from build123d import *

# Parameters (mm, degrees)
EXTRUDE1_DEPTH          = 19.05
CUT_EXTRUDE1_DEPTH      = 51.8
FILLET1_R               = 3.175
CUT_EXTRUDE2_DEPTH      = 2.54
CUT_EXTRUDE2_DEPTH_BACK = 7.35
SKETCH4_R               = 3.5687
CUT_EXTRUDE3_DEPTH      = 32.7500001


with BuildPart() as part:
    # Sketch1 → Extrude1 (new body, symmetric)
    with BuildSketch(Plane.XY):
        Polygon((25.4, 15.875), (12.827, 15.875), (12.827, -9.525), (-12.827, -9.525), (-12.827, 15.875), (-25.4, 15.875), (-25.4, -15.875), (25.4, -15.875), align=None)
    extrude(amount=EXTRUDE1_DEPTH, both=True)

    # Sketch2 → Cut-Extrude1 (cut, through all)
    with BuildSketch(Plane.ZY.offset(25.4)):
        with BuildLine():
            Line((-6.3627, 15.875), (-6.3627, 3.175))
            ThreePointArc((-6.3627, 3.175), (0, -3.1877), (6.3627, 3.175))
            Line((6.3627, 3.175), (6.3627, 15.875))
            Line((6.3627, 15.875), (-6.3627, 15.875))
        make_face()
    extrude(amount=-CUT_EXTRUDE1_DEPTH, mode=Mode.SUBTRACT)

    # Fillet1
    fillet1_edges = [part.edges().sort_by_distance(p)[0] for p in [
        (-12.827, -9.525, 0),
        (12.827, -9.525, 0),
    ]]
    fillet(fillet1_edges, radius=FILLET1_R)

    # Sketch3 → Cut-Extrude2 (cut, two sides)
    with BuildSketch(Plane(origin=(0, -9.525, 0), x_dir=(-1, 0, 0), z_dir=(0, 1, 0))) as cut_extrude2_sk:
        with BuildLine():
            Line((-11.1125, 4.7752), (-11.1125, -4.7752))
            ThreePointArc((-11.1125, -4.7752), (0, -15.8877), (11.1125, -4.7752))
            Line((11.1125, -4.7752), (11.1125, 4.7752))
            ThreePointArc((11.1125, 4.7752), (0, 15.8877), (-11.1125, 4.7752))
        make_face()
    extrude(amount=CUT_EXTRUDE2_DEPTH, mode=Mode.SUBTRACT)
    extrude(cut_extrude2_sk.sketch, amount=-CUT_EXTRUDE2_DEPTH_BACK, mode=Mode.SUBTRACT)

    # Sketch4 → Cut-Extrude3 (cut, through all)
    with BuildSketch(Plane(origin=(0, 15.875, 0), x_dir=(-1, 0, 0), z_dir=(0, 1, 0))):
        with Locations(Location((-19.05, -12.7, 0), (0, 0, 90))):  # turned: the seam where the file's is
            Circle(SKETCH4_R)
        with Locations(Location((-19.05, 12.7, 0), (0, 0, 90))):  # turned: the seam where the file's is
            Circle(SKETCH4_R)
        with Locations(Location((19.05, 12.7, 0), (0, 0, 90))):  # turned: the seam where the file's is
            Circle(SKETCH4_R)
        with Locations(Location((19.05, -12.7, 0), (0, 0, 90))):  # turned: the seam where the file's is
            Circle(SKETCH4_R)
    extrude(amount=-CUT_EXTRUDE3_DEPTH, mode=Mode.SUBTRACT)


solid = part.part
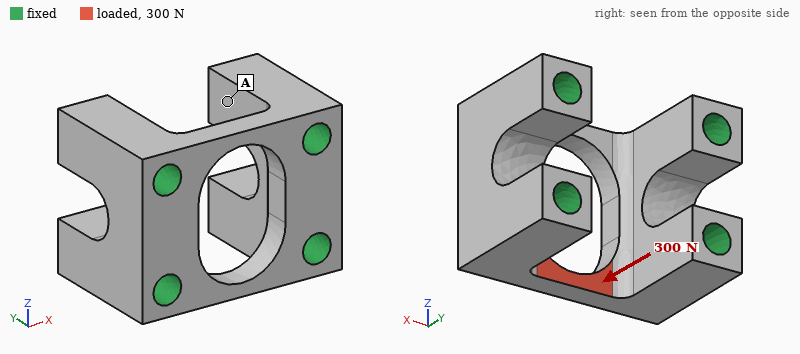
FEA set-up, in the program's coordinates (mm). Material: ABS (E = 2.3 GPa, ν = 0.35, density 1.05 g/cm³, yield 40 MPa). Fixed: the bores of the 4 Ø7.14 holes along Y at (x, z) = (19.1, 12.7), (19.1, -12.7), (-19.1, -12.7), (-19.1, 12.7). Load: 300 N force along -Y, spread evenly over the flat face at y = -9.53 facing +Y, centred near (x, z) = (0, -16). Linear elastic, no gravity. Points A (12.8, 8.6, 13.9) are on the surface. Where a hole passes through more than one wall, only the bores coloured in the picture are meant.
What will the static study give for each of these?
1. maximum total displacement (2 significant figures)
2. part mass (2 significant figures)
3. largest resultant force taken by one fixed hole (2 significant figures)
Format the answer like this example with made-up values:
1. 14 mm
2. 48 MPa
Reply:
1. 0.13 mm
2. 23 g
3. 150 N
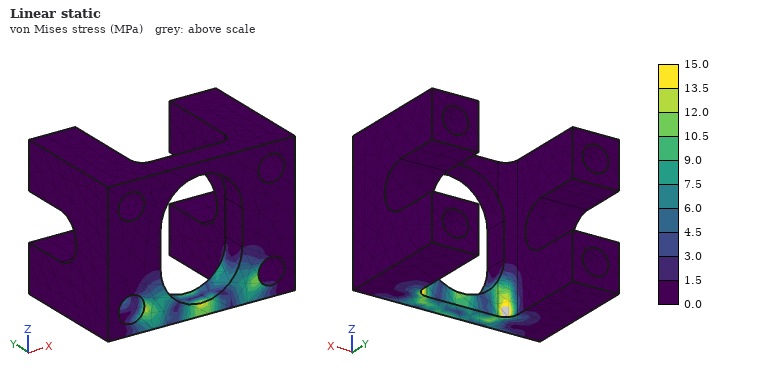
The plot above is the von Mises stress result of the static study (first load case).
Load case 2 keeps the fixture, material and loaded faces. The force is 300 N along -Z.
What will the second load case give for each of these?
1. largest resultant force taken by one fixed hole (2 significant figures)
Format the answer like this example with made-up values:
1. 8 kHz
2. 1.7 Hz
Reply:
1. 130 N
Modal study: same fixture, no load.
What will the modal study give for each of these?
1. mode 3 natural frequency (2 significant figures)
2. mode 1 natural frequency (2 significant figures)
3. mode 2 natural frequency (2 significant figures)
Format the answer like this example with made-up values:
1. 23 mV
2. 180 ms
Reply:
1. 14 kHz
2. 11 kHz
3. 11 kHz
